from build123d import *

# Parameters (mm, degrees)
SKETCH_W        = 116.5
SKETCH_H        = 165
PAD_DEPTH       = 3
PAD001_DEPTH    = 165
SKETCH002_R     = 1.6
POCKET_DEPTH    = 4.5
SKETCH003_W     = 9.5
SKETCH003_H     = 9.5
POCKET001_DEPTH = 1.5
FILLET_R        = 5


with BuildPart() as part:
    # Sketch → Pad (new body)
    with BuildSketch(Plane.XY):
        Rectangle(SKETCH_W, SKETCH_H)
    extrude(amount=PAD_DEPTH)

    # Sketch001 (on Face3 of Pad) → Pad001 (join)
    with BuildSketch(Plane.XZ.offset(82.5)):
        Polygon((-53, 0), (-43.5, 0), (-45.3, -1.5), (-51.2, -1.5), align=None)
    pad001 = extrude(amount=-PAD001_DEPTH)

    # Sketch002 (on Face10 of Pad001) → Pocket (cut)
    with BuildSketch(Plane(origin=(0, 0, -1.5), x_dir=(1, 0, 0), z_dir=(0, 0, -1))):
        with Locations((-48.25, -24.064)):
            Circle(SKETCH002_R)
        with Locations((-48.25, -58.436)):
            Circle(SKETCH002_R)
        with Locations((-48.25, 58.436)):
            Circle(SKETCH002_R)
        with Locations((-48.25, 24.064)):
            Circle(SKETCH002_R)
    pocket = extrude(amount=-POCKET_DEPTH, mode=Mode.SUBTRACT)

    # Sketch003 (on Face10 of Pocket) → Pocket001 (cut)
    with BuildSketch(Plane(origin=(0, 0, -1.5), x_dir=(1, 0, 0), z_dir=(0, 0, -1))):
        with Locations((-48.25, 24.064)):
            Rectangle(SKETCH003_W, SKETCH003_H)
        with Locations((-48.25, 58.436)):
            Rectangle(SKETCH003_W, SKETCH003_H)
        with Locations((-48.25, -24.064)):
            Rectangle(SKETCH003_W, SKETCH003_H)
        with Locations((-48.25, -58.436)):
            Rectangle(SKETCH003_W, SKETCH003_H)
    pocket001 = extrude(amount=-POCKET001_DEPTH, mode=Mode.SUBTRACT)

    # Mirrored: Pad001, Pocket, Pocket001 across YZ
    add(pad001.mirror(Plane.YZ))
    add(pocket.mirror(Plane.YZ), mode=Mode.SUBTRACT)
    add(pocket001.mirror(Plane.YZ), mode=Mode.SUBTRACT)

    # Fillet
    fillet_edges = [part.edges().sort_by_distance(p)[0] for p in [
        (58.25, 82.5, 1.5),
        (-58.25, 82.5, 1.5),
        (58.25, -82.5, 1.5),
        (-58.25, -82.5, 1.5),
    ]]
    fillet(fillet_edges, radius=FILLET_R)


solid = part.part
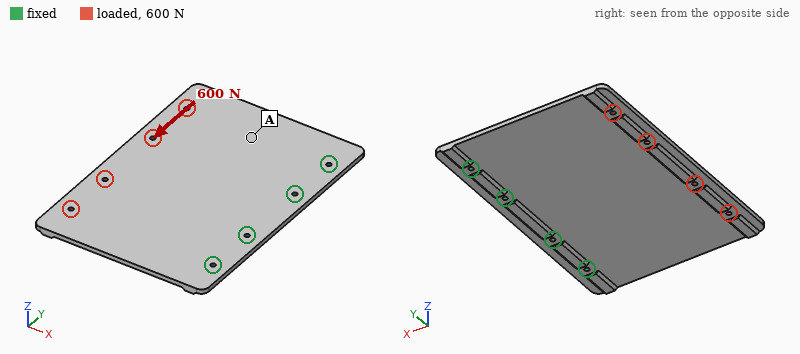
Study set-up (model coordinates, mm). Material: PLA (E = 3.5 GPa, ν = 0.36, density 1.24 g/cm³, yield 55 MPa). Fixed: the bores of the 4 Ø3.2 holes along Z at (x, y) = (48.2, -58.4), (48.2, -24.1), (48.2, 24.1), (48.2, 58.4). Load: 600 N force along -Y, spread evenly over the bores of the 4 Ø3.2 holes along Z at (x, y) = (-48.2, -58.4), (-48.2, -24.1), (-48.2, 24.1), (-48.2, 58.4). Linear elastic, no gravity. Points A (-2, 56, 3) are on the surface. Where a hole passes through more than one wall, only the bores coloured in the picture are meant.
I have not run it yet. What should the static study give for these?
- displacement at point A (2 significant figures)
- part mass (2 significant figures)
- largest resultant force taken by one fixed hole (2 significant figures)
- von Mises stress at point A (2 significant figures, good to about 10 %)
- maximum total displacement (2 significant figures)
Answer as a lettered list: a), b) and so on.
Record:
a) 0.13 mm
b) 75 g
c) 460 N
d) 2.1 MPa
e) 0.27 mm
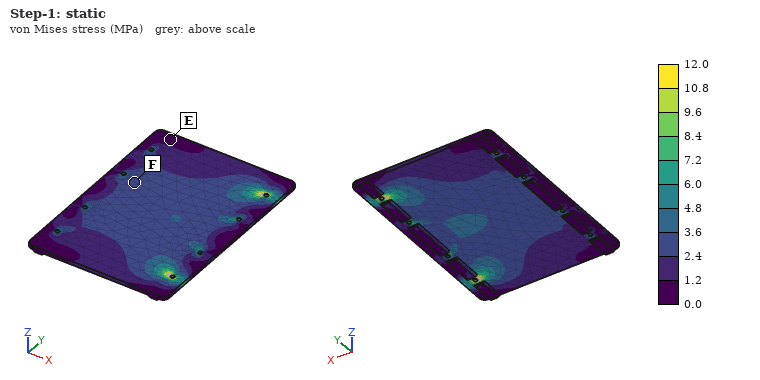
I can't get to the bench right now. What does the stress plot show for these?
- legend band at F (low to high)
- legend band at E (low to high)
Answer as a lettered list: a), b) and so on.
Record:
a) 2.4 to 3.6 MPa
b) 0.0 to 1.2 MPa
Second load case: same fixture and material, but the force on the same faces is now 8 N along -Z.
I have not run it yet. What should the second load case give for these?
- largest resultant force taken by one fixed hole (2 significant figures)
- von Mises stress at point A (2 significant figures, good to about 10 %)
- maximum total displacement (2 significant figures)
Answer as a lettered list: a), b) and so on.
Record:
a) 3.1 N
b) 1.4 MPa
c) 2.2 mm
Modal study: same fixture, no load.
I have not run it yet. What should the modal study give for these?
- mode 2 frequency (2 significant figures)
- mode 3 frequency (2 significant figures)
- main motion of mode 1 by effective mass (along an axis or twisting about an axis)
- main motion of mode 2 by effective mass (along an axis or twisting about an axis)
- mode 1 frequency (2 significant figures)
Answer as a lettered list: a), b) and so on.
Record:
a) 130 Hz
b) 290 Hz
c) along Z
d) twisting about X
e) 69 Hz
